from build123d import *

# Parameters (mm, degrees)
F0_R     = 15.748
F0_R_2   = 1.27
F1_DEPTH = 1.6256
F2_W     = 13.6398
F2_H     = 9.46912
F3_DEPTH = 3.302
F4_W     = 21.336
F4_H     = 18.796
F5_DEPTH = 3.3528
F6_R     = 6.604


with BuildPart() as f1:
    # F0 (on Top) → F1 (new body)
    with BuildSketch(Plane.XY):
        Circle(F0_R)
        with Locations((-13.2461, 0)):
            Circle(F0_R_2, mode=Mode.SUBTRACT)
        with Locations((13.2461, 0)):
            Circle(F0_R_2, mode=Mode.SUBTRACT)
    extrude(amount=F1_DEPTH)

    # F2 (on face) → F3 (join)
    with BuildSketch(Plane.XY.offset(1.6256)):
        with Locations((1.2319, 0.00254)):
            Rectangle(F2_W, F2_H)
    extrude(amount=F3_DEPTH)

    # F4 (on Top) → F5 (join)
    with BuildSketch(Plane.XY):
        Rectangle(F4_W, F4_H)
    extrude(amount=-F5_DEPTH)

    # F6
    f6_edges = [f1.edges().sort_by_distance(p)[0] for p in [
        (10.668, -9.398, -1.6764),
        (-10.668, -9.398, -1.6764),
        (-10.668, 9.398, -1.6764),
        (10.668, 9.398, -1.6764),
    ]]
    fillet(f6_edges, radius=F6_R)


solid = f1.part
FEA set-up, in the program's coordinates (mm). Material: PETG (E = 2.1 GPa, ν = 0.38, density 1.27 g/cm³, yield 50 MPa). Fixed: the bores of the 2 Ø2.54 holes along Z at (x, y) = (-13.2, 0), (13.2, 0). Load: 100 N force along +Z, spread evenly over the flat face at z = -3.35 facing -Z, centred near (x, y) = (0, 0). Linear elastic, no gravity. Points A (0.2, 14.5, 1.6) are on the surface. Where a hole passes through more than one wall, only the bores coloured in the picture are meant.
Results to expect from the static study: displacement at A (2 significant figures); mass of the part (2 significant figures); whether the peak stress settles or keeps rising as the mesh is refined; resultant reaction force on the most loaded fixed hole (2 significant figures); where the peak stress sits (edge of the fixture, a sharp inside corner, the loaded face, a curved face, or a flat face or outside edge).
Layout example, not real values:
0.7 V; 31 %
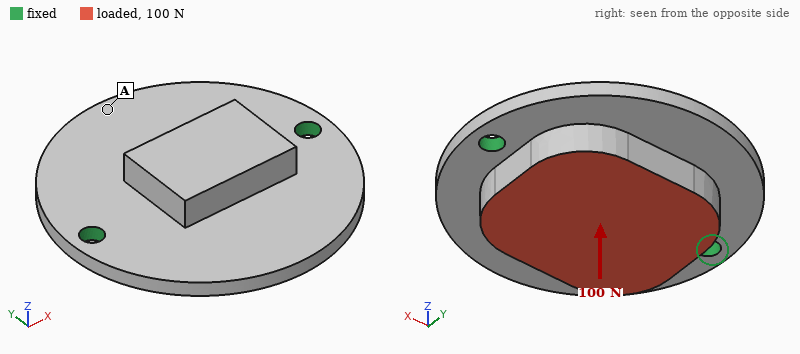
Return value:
75 µm; 3.7 g; keeps rising; 58 N; edge of the fixture
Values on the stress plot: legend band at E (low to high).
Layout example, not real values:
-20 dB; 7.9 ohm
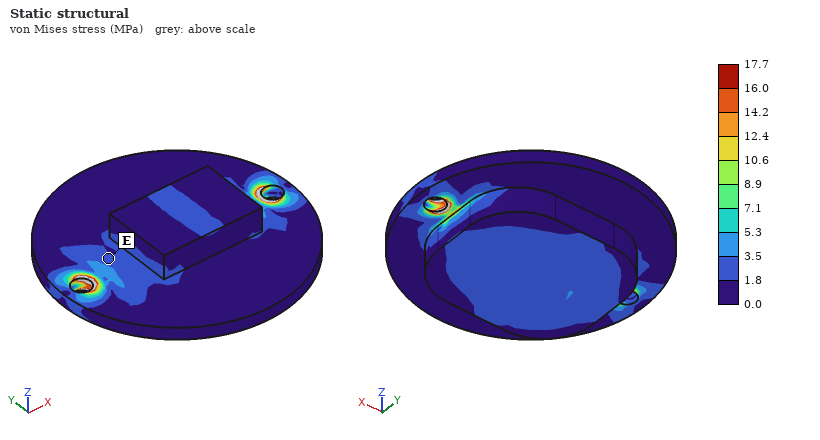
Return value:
1.8 to 3.5 MPa
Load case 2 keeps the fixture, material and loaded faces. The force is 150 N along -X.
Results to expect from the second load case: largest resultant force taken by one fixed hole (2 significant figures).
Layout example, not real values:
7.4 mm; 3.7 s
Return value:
81 N
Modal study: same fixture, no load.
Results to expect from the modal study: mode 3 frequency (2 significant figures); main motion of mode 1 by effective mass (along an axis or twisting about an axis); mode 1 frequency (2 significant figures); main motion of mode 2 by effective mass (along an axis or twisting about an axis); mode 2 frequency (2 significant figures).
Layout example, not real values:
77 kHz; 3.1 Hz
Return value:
6500 Hz; twisting about X; 1400 Hz; along Z; 3500 Hz
